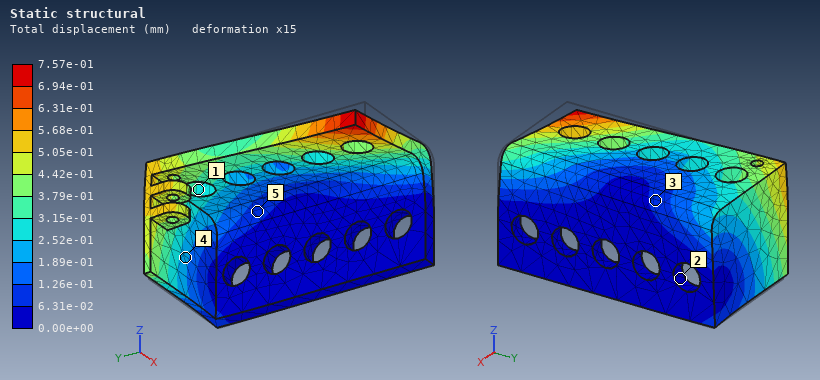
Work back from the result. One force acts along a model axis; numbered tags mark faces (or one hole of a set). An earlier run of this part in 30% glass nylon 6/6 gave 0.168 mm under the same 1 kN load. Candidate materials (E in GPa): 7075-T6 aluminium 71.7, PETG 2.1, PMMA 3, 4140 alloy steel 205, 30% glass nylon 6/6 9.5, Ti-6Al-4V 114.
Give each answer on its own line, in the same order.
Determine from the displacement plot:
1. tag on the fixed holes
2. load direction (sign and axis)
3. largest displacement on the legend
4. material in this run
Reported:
2
+Y
7.57e-01 mm
PETG
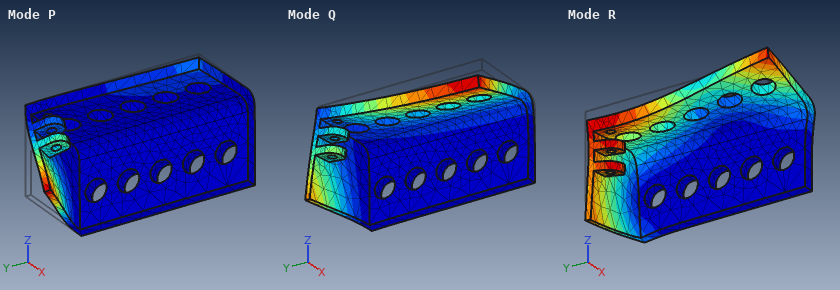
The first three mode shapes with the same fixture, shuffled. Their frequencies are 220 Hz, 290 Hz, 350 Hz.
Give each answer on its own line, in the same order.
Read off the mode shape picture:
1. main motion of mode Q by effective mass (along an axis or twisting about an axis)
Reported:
along Z
